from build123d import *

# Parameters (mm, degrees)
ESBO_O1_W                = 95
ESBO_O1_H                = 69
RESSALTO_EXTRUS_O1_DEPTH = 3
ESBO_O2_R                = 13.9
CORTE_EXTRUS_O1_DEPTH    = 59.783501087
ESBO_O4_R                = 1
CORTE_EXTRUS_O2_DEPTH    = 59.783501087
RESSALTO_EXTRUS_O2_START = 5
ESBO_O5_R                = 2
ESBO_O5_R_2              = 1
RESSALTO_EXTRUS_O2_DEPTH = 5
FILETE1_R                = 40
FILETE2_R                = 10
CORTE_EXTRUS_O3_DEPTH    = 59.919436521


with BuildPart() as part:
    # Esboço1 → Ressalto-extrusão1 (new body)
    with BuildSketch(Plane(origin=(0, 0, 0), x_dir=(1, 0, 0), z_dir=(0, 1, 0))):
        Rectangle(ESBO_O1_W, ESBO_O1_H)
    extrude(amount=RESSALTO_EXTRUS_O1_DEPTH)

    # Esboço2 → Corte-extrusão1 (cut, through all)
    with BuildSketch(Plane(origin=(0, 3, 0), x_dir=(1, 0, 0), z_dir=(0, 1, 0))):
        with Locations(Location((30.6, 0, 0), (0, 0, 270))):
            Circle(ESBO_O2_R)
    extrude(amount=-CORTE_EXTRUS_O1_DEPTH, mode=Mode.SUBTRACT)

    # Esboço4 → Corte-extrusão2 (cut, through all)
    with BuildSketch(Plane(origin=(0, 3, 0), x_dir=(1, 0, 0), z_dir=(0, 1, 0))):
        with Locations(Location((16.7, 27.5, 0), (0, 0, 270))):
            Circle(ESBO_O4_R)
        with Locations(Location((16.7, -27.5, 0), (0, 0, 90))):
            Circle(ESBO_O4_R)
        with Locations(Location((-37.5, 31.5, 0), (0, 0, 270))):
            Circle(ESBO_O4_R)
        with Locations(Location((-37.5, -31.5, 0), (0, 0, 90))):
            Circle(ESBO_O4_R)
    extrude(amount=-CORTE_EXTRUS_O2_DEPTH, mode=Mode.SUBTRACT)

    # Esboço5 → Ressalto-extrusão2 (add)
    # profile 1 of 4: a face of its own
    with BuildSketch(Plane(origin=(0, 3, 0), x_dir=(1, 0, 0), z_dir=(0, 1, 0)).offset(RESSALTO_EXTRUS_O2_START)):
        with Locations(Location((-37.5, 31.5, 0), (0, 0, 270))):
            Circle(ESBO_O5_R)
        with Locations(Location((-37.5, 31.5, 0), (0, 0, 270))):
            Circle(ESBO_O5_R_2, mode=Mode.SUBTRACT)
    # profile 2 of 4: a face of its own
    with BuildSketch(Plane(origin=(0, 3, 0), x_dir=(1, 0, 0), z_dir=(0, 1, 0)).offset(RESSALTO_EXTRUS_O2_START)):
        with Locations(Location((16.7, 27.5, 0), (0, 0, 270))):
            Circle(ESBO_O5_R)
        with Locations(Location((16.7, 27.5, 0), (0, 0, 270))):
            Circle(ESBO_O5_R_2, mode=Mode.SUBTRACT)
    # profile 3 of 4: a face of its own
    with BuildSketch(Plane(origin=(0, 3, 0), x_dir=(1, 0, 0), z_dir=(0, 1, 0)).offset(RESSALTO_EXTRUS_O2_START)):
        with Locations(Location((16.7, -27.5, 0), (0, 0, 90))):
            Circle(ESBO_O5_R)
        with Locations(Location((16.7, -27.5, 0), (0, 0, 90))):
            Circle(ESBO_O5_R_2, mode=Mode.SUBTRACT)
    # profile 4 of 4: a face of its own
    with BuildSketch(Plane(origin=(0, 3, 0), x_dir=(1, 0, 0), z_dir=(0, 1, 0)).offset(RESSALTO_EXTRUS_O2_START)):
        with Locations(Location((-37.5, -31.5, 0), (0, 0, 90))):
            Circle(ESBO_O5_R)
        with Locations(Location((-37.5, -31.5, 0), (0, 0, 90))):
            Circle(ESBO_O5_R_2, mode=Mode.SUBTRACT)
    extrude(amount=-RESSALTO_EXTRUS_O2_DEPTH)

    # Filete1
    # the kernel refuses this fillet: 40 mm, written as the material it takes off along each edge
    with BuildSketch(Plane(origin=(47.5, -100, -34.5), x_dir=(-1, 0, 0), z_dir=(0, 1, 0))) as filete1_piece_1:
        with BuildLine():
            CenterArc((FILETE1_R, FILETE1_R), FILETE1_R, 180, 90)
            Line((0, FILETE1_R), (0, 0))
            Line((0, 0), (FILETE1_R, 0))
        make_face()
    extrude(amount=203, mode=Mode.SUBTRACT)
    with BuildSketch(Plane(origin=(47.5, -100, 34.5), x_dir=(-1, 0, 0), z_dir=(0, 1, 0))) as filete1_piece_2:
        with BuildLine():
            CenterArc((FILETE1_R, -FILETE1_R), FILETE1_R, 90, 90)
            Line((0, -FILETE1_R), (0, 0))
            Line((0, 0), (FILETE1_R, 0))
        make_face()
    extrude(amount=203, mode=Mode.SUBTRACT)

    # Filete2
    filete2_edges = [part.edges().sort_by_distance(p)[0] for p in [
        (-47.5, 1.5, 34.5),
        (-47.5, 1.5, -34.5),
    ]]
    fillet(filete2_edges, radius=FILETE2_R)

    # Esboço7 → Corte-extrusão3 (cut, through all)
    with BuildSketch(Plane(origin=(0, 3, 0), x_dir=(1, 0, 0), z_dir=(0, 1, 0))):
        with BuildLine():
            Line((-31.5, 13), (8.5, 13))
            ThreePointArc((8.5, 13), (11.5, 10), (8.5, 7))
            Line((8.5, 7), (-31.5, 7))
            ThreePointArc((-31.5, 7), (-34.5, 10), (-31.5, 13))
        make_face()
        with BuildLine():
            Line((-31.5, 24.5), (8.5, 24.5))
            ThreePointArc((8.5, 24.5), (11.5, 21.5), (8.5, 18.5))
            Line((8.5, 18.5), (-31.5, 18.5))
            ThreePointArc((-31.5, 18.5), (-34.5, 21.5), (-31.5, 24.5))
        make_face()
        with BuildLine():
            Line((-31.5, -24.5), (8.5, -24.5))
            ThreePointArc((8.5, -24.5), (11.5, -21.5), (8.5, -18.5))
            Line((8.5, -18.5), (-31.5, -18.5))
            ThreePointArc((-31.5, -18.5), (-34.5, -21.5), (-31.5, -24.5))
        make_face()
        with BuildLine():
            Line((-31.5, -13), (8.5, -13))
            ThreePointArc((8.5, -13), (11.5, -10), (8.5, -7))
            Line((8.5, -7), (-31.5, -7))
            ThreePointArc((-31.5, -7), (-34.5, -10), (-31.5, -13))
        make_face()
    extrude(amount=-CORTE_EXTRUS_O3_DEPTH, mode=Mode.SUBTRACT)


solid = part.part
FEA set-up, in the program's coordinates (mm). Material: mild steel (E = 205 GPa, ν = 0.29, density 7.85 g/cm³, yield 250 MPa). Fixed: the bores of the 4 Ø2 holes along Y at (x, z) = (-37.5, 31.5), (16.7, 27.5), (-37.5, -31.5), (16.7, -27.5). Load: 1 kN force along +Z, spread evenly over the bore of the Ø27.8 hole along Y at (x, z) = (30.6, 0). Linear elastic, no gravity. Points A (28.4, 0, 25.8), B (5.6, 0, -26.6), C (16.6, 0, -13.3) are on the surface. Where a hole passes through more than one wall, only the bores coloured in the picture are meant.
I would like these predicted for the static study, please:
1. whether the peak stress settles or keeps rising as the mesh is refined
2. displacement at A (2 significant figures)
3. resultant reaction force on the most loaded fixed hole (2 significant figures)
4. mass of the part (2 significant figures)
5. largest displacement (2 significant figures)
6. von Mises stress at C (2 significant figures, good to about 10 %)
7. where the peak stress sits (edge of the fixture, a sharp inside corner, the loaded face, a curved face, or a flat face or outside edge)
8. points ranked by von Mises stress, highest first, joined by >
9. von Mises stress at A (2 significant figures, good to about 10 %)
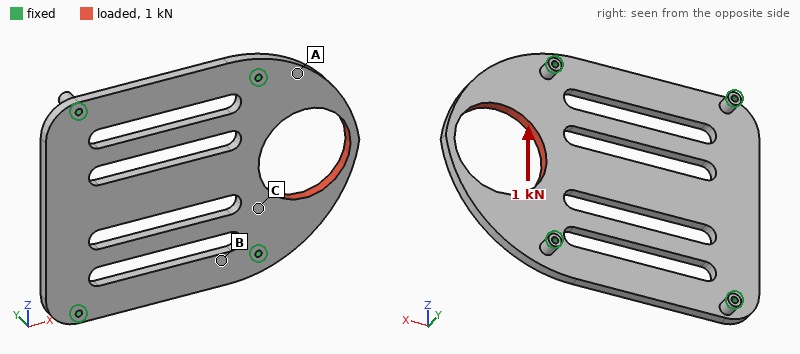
keeps rising
2.9 µm
550 N
99 g
12 µm
11 MPa
edge of the fixture
A > C > B
17 MPa
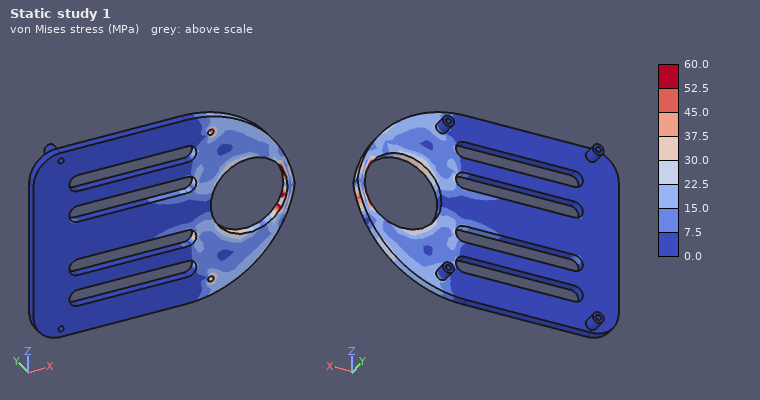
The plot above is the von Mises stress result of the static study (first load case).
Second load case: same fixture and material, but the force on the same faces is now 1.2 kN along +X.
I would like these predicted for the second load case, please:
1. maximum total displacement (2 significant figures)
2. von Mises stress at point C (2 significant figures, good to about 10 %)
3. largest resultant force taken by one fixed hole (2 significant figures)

4.5 µm
6.7 MPa
520 N
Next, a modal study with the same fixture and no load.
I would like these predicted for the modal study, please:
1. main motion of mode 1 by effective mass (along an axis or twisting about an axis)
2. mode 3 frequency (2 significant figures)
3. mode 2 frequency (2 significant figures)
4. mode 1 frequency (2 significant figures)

along Y
4100 Hz
3100 Hz
2500 Hz
